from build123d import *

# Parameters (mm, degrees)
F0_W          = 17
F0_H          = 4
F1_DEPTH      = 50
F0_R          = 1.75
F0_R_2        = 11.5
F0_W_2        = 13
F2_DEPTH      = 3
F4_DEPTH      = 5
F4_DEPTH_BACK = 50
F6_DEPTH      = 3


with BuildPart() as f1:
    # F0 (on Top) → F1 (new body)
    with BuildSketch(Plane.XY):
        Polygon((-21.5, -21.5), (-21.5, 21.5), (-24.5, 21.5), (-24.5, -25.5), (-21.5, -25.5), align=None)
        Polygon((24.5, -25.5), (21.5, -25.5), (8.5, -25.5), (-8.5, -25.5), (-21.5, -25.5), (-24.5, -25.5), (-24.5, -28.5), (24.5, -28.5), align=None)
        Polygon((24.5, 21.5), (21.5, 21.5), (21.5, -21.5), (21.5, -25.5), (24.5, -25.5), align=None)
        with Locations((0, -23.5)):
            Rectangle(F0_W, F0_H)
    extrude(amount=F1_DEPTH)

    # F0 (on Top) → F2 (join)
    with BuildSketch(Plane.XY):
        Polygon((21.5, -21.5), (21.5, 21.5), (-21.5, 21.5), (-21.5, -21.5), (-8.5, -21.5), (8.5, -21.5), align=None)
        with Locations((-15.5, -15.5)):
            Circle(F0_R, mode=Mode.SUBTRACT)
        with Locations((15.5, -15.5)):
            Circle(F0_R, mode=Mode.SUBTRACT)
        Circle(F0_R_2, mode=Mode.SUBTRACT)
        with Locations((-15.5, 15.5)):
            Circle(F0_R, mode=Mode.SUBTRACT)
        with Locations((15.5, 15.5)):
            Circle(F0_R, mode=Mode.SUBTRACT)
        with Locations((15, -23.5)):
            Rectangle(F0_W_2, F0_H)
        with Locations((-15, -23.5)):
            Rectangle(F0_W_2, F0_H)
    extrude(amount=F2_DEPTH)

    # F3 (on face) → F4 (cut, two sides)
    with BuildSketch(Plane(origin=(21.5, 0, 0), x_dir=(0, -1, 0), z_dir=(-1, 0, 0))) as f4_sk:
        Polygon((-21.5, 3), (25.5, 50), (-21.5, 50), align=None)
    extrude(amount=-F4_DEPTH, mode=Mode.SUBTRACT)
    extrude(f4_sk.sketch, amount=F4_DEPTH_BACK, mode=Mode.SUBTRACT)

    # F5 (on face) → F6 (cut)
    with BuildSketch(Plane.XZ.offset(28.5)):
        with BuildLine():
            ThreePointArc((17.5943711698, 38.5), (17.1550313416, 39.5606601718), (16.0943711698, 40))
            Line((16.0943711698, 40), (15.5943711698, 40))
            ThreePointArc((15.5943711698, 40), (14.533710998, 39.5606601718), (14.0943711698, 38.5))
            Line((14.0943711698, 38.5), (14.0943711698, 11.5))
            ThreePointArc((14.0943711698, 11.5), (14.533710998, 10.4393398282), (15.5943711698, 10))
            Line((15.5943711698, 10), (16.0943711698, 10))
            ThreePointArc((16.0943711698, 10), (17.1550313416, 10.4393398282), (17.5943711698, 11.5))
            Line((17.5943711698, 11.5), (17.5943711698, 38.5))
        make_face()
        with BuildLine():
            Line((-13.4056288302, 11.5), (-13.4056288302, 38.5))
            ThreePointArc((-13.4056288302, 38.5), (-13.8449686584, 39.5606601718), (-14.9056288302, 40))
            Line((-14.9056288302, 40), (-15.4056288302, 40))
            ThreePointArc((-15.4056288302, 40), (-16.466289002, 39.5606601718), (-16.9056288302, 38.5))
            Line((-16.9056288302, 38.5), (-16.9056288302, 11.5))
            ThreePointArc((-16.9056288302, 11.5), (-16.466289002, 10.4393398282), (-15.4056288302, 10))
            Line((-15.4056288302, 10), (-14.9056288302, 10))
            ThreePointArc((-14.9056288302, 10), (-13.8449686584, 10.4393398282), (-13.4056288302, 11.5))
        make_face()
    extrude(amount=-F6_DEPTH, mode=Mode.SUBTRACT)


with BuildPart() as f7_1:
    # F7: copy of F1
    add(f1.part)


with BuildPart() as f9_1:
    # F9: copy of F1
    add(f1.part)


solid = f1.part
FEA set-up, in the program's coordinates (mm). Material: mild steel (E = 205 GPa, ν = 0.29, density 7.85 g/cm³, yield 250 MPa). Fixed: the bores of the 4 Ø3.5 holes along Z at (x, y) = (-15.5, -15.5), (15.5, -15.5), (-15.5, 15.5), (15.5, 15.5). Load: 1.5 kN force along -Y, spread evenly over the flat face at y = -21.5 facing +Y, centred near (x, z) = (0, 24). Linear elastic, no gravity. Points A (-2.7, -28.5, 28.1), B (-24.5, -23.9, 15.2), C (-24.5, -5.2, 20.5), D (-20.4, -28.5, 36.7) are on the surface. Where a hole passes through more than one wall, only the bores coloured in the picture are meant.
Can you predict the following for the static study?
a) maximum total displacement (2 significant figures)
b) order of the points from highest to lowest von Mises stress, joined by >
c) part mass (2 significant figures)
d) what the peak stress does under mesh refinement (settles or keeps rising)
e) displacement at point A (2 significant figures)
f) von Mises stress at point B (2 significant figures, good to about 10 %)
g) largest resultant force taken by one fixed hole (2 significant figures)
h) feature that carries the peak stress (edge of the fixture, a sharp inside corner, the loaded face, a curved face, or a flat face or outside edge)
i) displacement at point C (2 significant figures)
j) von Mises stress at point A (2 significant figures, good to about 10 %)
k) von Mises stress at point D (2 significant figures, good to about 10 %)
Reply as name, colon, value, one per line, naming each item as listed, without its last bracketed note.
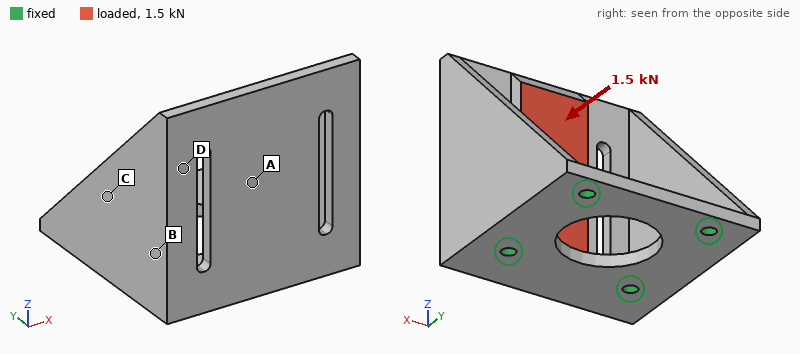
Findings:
maximum total displacement: 83 µm
order of the points from highest to lowest von Mises stress, joined by >: D > B > A > C
part mass: 170 g
what the peak stress does under mesh refinement: keeps rising
displacement at point A: 53 µm
von Mises stress at point B: 39 MPa
largest resultant force taken by one fixed hole: 780 N
feature that carries the peak stress: edge of the fixture
displacement at point C: 20 µm
von Mises stress at point A: 23 MPa
von Mises stress at point D: 60 MPa
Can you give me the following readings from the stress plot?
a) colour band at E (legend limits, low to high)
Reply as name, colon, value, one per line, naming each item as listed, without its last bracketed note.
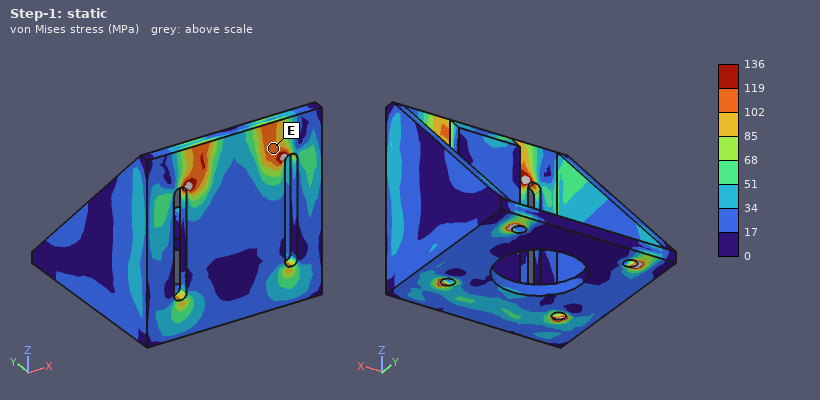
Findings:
colour band at E: 102 to 119 MPa
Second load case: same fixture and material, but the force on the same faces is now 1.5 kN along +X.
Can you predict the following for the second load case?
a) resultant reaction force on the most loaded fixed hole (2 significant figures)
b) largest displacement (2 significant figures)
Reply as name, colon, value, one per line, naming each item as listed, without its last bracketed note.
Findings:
resultant reaction force on the most loaded fixed hole: 1.4 kN
largest displacement: 49 µm
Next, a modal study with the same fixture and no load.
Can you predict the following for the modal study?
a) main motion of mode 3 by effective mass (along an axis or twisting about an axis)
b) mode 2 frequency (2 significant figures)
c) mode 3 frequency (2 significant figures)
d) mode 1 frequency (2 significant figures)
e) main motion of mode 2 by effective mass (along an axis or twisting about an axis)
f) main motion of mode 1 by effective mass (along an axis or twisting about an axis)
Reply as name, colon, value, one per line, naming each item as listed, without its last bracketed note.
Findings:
main motion of mode 3 by effective mass: along Z
mode 2 frequency: 3100 Hz
mode 3 frequency: 5400 Hz
mode 1 frequency: 2900 Hz
main motion of mode 2 by effective mass: along X
main motion of mode 1 by effective mass: along Y
